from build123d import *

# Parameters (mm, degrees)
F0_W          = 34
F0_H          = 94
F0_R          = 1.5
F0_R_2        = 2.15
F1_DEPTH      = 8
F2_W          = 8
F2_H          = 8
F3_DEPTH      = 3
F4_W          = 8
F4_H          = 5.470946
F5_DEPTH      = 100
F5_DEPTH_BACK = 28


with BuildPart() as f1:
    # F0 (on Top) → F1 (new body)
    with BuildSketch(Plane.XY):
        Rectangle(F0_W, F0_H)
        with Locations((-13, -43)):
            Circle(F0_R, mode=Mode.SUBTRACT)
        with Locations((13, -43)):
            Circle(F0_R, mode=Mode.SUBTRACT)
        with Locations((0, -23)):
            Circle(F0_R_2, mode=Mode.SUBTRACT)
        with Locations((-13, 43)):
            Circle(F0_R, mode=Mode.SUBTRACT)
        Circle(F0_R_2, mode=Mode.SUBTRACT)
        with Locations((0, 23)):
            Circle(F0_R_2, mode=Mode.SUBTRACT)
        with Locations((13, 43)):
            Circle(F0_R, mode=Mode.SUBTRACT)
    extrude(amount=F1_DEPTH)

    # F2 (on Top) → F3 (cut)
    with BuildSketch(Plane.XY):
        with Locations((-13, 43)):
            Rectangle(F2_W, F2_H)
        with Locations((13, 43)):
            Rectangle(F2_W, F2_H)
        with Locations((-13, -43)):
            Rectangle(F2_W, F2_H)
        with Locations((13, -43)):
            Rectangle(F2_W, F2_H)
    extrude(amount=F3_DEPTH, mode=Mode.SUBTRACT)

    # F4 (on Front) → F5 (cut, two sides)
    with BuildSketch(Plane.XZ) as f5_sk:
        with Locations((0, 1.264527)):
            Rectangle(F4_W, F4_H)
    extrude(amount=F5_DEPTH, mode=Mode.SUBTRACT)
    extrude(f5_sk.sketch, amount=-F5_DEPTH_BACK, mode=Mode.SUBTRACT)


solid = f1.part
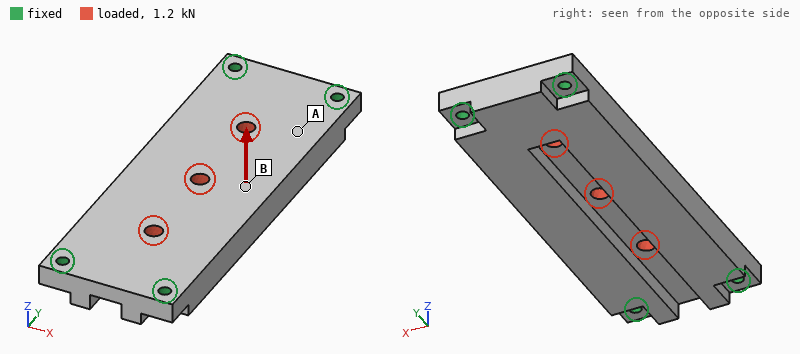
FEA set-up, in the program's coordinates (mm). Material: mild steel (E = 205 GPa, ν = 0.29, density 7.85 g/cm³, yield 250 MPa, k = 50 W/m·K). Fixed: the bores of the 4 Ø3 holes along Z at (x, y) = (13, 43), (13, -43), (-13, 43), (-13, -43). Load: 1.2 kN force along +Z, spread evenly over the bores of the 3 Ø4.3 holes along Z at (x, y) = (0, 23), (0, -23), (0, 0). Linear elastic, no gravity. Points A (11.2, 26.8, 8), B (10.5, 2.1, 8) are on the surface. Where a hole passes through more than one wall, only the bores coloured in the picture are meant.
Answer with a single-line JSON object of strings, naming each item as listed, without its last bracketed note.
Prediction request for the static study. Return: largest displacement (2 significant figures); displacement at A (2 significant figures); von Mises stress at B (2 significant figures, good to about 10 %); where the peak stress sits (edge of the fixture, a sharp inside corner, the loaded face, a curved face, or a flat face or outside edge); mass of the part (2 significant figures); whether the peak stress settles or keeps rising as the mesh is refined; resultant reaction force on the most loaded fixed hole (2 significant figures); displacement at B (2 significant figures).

{"largest displacement": "22 µm", "displacement at A": "9.4 µm", "von Mises stress at B": "22 MPa", "where the peak stress sits": "edge of the fixture", "mass of the part": "170 g", "whether the peak stress settles or keeps rising as the mesh is refined": "keeps rising", "resultant reaction force on the most loaded fixed hole": "440 N", "displacement at B": "19 µm"}
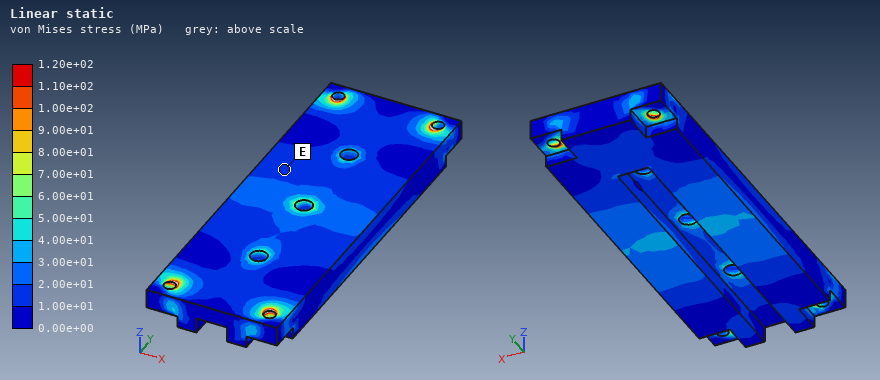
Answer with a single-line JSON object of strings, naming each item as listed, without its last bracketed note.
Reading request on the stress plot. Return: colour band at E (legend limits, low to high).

{"colour band at E": "1.00e+01 to 2.00e+01 MPa"}
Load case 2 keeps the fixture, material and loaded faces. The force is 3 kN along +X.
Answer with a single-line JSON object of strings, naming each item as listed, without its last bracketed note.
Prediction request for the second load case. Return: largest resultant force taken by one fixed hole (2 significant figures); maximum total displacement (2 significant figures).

{"largest resultant force taken by one fixed hole": "1.2 kN", "maximum total displacement": "5.8 µm"}
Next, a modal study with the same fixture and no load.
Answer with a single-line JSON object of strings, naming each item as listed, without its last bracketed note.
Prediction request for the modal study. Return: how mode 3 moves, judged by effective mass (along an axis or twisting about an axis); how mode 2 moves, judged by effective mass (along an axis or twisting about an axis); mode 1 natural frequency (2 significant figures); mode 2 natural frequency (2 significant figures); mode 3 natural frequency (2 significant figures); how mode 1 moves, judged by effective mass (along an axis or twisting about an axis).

{"how mode 3 moves, judged by effective mass": "twisting about X", "how mode 2 moves, judged by effective mass": "twisting about Y", "mode 1 natural frequency": "4000 Hz", "mode 2 natural frequency": "7700 Hz", "mode 3 natural frequency": "11 kHz", "how mode 1 moves, judged by effective mass": "along Z"}
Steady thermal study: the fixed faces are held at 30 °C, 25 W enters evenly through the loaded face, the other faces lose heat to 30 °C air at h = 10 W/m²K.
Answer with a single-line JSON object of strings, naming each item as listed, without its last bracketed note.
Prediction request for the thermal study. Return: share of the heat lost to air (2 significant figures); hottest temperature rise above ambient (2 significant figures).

{"share of the heat lost to air": "7.1 %", "hottest temperature rise above ambient": "40 K"}
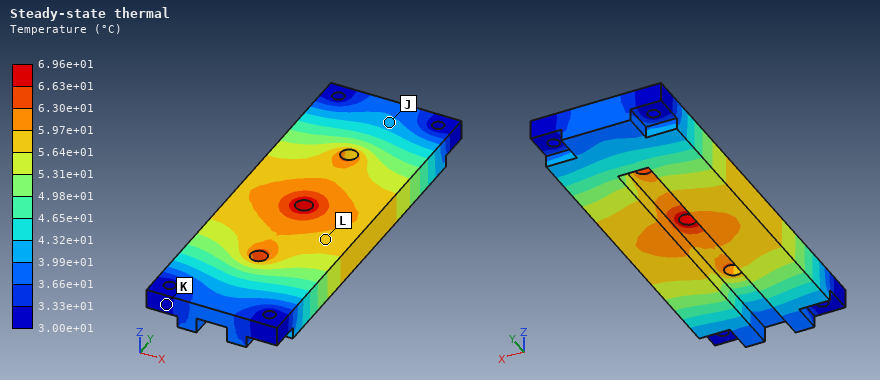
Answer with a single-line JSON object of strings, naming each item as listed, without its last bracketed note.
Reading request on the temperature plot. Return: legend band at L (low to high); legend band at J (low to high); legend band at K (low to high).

{"legend band at L": "5.64e+01 to 5.97e+01 °C", "legend band at J": "3.99e+01 to 4.32e+01 °C", "legend band at K": "3.00e+01 to 3.33e+01 °C"}
